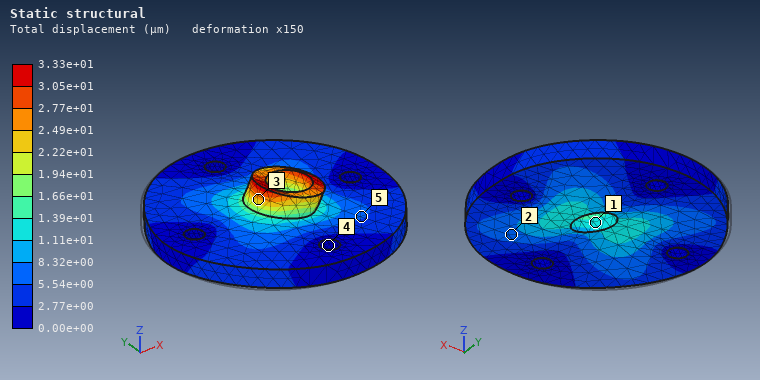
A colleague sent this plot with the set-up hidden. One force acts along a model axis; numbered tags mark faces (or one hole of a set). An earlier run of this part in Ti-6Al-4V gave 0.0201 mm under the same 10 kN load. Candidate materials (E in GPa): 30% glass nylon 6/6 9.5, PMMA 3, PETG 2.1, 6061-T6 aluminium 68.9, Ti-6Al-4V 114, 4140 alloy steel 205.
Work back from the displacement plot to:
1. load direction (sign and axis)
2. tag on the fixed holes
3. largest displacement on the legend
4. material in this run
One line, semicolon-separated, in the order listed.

+X; 4; 3.33e+01 µm; 6061-T6 aluminium
